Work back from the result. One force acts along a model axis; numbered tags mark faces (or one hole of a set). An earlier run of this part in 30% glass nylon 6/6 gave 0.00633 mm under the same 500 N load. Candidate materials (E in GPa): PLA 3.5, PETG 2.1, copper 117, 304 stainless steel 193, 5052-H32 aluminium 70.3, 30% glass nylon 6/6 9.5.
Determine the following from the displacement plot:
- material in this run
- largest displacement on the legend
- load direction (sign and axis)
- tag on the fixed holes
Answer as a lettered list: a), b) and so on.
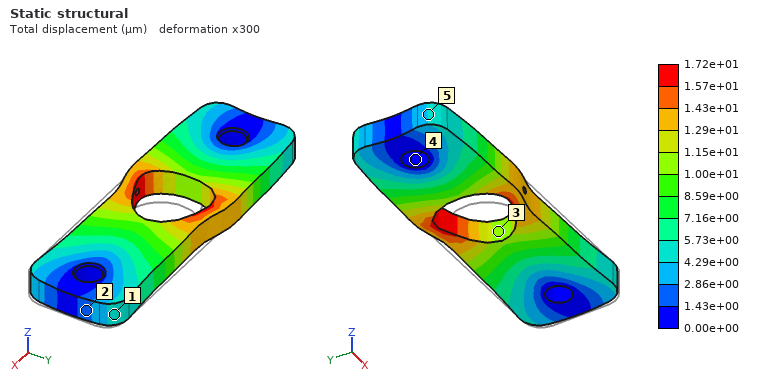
a) PLA
b) 1.72e+01 µm
c) -X
d) 4
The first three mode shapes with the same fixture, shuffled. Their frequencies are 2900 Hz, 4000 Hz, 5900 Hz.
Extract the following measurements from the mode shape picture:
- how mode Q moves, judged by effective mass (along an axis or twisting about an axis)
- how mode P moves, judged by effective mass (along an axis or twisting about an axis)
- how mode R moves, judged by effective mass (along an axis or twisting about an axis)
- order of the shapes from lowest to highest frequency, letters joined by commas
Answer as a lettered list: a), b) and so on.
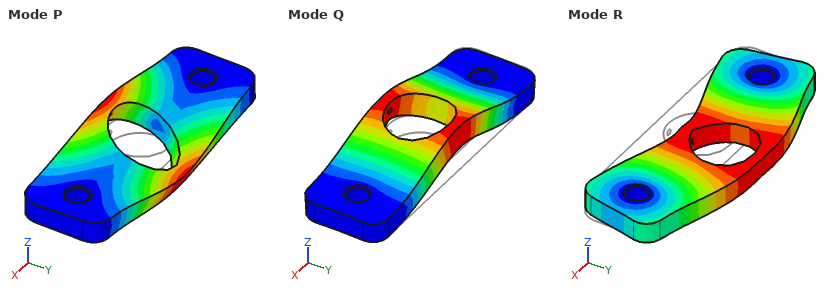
a) along Z
b) twisting about X
c) along Y
d) Q, P, R
